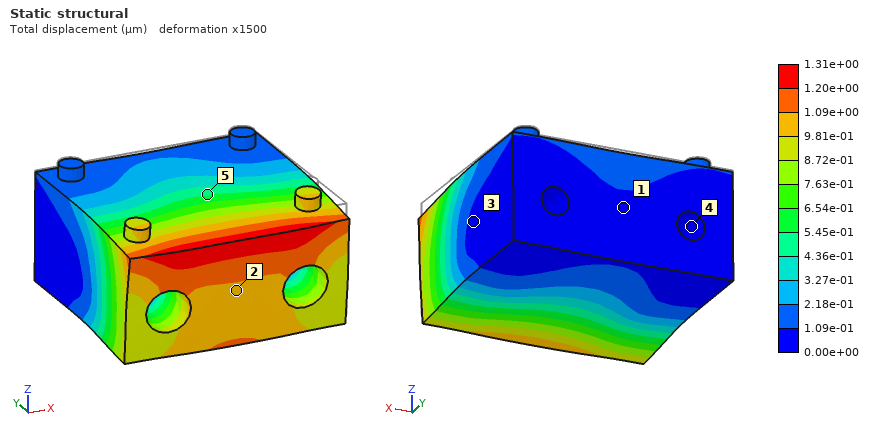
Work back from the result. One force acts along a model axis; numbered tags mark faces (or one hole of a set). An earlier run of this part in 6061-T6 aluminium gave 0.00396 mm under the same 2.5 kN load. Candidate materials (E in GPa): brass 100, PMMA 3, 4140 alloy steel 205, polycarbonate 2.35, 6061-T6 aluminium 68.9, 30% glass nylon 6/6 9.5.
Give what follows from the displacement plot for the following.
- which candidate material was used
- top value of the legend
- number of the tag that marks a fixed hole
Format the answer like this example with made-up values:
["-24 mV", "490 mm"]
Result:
["4140 alloy steel", "1.31e+00 µm", "4"]
